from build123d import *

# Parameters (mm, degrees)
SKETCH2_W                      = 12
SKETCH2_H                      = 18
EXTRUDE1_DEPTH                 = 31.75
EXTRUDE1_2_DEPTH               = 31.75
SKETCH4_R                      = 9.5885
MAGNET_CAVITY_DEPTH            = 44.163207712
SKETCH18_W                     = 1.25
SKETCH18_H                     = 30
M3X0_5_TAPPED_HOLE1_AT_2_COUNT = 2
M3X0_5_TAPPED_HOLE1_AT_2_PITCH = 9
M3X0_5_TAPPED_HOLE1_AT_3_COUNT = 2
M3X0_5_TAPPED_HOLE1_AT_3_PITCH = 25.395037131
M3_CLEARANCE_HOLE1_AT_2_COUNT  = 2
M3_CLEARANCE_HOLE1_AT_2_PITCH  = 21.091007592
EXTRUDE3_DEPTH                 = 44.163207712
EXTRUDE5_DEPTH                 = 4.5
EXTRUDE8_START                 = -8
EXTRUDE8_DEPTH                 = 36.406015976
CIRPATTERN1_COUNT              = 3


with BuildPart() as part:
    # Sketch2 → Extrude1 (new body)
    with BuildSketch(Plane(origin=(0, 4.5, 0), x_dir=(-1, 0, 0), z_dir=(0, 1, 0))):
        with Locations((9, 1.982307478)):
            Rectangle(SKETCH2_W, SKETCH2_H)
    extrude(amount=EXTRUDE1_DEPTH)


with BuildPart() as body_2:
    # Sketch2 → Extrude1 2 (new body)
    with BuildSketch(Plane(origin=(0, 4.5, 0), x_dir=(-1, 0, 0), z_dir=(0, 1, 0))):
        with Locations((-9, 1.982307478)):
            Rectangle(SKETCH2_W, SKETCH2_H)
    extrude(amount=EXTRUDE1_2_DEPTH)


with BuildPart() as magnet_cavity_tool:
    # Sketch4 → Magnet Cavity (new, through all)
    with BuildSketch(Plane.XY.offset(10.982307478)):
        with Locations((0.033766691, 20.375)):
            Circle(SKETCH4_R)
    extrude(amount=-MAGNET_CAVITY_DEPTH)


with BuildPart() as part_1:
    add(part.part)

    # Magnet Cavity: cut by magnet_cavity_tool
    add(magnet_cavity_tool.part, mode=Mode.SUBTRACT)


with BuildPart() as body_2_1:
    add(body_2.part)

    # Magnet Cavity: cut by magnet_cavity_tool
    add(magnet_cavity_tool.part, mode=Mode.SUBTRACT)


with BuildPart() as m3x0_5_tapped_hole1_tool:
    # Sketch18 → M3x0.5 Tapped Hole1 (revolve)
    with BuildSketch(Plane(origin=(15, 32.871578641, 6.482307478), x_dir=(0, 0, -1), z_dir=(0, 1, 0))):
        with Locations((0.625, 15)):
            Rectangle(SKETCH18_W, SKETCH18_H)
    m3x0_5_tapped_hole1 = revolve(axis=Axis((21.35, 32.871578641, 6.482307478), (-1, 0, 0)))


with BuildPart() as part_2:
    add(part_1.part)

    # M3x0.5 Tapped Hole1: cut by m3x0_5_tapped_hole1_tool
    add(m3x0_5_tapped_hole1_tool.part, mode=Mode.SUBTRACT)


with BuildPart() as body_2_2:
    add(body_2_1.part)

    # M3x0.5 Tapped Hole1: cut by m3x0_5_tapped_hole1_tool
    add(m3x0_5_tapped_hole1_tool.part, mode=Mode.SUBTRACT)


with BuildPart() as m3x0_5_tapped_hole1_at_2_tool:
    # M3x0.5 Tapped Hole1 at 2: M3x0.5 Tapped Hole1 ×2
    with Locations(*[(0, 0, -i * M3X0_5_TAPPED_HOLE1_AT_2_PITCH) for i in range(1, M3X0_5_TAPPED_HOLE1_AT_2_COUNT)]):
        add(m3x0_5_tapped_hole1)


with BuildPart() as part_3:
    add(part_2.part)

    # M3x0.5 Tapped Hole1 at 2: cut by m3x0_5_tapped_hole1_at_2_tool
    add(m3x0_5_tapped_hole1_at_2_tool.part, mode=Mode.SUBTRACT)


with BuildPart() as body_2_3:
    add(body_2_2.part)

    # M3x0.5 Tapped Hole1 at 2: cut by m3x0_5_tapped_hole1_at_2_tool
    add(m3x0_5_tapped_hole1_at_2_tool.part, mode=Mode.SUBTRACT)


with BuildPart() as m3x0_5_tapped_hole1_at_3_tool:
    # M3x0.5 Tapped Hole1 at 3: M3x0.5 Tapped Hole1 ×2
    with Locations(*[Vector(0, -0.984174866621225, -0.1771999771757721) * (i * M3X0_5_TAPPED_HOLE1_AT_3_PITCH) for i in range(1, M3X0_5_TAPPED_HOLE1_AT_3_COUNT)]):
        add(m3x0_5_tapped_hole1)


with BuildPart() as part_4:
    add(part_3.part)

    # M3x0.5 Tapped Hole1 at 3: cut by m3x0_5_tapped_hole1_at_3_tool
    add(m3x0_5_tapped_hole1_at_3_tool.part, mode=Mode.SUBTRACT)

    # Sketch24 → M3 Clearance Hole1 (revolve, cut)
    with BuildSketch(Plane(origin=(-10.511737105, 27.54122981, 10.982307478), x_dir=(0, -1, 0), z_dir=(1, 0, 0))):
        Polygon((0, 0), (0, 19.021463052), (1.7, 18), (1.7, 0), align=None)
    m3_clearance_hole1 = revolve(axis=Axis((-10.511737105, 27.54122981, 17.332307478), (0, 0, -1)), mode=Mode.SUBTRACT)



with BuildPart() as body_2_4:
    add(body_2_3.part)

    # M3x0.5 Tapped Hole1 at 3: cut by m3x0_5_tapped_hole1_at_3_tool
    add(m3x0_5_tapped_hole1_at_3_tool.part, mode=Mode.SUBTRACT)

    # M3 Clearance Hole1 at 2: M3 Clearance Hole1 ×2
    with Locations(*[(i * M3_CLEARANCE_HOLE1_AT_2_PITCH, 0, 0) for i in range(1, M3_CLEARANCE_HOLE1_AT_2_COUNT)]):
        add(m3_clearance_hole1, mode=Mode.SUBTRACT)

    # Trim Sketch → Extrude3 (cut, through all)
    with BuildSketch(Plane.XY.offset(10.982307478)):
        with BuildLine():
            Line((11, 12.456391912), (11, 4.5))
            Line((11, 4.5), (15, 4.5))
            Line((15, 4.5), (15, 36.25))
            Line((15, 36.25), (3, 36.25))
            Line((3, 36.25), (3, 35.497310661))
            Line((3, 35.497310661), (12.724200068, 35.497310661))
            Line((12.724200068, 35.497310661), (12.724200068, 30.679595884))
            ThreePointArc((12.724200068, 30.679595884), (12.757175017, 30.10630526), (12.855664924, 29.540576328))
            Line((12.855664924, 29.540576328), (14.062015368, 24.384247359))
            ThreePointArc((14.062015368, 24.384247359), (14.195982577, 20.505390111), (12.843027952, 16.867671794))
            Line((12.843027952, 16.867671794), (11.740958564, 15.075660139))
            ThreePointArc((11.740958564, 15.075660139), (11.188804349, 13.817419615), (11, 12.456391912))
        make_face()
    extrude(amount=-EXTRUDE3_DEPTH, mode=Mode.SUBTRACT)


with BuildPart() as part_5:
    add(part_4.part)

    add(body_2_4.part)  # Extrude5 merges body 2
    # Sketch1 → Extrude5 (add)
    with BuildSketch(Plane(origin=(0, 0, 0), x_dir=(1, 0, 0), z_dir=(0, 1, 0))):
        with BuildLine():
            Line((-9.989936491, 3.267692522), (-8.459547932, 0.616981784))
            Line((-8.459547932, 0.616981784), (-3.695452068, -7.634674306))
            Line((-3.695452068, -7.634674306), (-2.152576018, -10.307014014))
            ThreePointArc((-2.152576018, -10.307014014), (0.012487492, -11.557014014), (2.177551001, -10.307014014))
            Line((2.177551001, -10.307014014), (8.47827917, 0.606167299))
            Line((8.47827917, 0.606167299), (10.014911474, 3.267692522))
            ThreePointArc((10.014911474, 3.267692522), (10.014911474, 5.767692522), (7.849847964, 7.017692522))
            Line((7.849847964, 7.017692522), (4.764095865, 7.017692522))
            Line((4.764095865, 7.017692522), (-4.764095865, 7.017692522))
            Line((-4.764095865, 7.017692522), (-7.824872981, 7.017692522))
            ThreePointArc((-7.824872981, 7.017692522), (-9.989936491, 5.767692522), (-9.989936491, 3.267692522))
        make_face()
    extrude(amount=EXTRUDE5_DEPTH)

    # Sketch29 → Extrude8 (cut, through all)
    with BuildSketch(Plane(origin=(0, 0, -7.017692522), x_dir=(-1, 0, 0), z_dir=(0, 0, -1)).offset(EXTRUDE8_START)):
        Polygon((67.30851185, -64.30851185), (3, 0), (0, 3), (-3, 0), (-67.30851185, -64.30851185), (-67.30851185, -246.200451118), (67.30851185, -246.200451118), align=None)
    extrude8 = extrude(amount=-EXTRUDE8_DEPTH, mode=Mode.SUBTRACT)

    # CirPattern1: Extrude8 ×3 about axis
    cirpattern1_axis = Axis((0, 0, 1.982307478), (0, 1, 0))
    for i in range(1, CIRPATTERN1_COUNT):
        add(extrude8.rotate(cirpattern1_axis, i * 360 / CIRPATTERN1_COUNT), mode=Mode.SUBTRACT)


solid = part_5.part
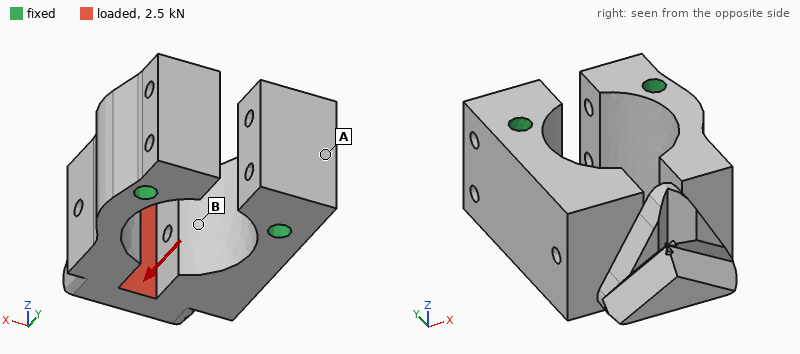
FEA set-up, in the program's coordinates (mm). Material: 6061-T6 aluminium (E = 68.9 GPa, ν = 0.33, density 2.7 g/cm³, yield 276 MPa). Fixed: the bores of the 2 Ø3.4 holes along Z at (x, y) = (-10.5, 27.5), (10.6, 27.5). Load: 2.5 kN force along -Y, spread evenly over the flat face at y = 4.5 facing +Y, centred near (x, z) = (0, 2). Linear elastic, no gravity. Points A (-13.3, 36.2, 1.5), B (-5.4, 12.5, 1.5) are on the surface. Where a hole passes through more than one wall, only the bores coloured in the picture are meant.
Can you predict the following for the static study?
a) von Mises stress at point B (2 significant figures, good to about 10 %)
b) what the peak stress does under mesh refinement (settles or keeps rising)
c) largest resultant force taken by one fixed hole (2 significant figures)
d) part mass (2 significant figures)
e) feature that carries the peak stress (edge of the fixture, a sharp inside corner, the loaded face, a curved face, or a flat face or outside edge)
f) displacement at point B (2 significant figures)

21 MPa
keeps rising
1.4 kN
25 g
a sharp inside corner
8.8 µm
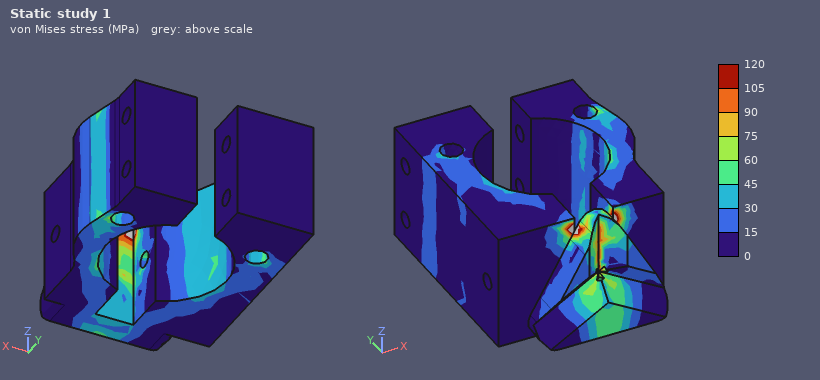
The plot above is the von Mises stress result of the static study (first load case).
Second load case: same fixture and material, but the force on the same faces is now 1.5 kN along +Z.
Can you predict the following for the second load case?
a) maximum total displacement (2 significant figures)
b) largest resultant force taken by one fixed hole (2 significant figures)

45 µm
760 N
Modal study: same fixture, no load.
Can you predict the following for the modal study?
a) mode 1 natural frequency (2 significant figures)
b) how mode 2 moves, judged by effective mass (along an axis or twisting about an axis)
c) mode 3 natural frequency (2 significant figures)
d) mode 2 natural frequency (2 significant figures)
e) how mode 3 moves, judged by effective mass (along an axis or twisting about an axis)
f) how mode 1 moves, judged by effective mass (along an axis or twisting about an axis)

9900 Hz
along Z
19 kHz
12 kHz
twisting about Y
along X
